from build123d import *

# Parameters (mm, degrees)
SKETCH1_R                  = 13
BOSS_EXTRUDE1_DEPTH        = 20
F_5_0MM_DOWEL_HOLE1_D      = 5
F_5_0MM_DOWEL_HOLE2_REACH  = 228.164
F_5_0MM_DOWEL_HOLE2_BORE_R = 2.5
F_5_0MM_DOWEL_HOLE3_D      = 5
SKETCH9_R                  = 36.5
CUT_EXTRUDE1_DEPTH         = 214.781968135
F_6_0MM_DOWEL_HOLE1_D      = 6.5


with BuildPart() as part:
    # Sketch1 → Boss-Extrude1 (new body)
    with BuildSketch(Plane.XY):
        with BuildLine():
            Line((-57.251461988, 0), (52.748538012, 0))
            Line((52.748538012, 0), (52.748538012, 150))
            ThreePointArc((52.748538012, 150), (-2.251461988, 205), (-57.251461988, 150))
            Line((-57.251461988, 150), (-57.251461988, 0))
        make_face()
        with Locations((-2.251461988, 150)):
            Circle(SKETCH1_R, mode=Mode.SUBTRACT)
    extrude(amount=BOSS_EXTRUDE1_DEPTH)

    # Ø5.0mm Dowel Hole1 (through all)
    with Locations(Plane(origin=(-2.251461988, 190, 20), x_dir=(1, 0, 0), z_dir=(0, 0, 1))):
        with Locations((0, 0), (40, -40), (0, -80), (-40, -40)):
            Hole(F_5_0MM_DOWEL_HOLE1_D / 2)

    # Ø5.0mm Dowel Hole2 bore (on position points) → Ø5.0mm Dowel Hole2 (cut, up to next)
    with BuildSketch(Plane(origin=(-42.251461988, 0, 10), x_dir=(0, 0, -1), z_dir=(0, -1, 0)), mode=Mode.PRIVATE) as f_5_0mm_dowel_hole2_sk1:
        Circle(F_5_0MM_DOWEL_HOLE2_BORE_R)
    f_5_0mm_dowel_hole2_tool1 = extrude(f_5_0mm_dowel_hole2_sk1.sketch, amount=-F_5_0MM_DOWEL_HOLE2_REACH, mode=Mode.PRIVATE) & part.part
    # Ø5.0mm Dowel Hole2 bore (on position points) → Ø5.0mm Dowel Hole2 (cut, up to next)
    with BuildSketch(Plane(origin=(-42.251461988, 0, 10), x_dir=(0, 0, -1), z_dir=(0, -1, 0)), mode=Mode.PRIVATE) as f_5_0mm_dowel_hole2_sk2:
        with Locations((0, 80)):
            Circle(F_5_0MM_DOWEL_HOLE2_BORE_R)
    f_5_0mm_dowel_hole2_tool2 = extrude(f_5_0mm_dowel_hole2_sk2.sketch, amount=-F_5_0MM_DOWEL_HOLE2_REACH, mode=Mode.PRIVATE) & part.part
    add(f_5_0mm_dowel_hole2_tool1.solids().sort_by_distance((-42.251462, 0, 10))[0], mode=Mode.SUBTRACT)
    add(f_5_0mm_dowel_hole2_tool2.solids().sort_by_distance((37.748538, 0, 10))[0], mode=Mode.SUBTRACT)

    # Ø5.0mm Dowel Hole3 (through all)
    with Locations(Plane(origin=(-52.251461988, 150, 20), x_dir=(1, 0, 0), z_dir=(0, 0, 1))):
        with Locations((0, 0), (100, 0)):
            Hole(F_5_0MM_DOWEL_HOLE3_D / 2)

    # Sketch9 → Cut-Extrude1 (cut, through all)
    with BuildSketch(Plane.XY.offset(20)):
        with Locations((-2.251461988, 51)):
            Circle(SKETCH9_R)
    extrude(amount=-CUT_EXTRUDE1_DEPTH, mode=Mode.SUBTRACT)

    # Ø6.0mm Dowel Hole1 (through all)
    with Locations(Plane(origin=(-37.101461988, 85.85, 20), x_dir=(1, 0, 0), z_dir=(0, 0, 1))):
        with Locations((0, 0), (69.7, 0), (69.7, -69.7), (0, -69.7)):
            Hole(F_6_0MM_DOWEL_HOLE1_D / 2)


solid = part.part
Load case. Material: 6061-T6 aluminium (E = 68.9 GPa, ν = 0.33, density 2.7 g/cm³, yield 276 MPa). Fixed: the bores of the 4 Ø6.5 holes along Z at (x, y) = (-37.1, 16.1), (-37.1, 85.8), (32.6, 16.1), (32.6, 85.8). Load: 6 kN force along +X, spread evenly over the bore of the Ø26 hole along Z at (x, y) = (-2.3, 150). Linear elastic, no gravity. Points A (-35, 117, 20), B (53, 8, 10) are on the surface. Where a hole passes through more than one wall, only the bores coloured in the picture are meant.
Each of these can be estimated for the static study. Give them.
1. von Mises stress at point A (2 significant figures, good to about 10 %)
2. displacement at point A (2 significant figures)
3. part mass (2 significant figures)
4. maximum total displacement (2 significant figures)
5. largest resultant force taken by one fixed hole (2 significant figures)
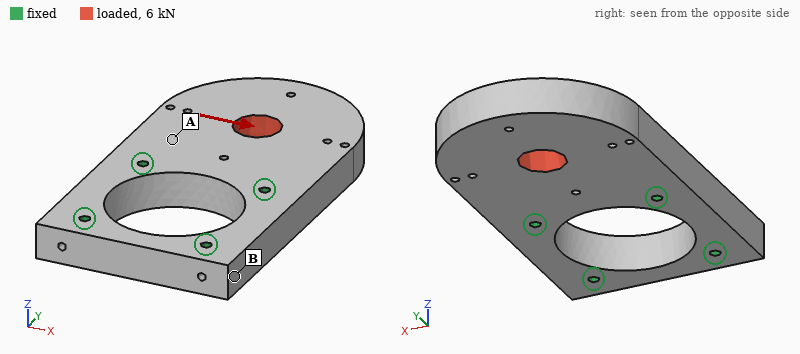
5.6 MPa
7.4 µm
860 g
23 µm
5.3 kN
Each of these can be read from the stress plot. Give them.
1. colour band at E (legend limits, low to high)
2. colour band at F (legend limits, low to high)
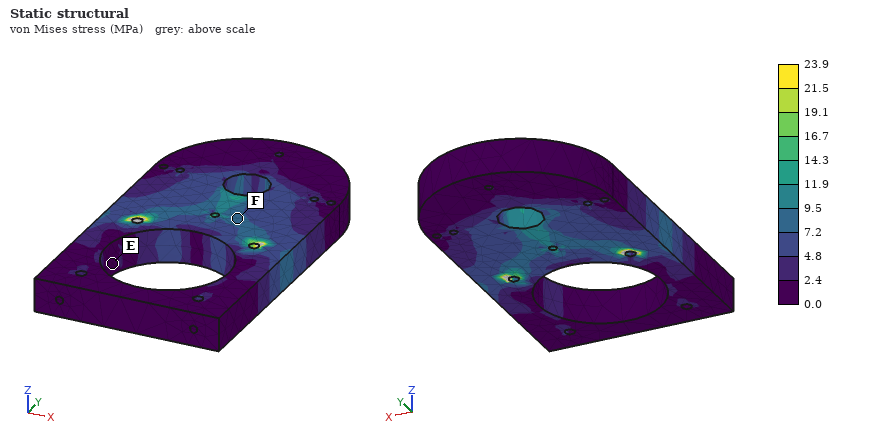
0.0 to 2.4 MPa
7.2 to 9.5 MPa
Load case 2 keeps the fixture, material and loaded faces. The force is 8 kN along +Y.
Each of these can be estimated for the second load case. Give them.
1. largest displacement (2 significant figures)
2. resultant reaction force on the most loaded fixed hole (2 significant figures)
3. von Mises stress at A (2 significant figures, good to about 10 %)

7.7 µm
3.9 kN
5.0 MPa
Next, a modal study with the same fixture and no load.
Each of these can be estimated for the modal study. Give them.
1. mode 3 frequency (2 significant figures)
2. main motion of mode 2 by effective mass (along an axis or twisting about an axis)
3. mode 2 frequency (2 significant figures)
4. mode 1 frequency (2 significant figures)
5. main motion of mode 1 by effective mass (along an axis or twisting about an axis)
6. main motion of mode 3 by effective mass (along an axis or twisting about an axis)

4200 Hz
twisting about Y
3200 Hz
1100 Hz
along Z
along X
